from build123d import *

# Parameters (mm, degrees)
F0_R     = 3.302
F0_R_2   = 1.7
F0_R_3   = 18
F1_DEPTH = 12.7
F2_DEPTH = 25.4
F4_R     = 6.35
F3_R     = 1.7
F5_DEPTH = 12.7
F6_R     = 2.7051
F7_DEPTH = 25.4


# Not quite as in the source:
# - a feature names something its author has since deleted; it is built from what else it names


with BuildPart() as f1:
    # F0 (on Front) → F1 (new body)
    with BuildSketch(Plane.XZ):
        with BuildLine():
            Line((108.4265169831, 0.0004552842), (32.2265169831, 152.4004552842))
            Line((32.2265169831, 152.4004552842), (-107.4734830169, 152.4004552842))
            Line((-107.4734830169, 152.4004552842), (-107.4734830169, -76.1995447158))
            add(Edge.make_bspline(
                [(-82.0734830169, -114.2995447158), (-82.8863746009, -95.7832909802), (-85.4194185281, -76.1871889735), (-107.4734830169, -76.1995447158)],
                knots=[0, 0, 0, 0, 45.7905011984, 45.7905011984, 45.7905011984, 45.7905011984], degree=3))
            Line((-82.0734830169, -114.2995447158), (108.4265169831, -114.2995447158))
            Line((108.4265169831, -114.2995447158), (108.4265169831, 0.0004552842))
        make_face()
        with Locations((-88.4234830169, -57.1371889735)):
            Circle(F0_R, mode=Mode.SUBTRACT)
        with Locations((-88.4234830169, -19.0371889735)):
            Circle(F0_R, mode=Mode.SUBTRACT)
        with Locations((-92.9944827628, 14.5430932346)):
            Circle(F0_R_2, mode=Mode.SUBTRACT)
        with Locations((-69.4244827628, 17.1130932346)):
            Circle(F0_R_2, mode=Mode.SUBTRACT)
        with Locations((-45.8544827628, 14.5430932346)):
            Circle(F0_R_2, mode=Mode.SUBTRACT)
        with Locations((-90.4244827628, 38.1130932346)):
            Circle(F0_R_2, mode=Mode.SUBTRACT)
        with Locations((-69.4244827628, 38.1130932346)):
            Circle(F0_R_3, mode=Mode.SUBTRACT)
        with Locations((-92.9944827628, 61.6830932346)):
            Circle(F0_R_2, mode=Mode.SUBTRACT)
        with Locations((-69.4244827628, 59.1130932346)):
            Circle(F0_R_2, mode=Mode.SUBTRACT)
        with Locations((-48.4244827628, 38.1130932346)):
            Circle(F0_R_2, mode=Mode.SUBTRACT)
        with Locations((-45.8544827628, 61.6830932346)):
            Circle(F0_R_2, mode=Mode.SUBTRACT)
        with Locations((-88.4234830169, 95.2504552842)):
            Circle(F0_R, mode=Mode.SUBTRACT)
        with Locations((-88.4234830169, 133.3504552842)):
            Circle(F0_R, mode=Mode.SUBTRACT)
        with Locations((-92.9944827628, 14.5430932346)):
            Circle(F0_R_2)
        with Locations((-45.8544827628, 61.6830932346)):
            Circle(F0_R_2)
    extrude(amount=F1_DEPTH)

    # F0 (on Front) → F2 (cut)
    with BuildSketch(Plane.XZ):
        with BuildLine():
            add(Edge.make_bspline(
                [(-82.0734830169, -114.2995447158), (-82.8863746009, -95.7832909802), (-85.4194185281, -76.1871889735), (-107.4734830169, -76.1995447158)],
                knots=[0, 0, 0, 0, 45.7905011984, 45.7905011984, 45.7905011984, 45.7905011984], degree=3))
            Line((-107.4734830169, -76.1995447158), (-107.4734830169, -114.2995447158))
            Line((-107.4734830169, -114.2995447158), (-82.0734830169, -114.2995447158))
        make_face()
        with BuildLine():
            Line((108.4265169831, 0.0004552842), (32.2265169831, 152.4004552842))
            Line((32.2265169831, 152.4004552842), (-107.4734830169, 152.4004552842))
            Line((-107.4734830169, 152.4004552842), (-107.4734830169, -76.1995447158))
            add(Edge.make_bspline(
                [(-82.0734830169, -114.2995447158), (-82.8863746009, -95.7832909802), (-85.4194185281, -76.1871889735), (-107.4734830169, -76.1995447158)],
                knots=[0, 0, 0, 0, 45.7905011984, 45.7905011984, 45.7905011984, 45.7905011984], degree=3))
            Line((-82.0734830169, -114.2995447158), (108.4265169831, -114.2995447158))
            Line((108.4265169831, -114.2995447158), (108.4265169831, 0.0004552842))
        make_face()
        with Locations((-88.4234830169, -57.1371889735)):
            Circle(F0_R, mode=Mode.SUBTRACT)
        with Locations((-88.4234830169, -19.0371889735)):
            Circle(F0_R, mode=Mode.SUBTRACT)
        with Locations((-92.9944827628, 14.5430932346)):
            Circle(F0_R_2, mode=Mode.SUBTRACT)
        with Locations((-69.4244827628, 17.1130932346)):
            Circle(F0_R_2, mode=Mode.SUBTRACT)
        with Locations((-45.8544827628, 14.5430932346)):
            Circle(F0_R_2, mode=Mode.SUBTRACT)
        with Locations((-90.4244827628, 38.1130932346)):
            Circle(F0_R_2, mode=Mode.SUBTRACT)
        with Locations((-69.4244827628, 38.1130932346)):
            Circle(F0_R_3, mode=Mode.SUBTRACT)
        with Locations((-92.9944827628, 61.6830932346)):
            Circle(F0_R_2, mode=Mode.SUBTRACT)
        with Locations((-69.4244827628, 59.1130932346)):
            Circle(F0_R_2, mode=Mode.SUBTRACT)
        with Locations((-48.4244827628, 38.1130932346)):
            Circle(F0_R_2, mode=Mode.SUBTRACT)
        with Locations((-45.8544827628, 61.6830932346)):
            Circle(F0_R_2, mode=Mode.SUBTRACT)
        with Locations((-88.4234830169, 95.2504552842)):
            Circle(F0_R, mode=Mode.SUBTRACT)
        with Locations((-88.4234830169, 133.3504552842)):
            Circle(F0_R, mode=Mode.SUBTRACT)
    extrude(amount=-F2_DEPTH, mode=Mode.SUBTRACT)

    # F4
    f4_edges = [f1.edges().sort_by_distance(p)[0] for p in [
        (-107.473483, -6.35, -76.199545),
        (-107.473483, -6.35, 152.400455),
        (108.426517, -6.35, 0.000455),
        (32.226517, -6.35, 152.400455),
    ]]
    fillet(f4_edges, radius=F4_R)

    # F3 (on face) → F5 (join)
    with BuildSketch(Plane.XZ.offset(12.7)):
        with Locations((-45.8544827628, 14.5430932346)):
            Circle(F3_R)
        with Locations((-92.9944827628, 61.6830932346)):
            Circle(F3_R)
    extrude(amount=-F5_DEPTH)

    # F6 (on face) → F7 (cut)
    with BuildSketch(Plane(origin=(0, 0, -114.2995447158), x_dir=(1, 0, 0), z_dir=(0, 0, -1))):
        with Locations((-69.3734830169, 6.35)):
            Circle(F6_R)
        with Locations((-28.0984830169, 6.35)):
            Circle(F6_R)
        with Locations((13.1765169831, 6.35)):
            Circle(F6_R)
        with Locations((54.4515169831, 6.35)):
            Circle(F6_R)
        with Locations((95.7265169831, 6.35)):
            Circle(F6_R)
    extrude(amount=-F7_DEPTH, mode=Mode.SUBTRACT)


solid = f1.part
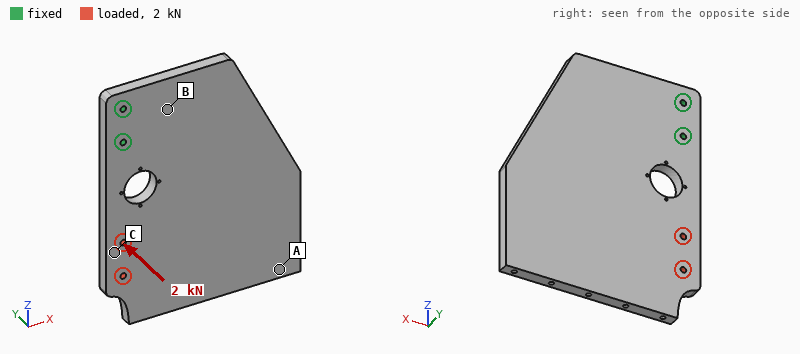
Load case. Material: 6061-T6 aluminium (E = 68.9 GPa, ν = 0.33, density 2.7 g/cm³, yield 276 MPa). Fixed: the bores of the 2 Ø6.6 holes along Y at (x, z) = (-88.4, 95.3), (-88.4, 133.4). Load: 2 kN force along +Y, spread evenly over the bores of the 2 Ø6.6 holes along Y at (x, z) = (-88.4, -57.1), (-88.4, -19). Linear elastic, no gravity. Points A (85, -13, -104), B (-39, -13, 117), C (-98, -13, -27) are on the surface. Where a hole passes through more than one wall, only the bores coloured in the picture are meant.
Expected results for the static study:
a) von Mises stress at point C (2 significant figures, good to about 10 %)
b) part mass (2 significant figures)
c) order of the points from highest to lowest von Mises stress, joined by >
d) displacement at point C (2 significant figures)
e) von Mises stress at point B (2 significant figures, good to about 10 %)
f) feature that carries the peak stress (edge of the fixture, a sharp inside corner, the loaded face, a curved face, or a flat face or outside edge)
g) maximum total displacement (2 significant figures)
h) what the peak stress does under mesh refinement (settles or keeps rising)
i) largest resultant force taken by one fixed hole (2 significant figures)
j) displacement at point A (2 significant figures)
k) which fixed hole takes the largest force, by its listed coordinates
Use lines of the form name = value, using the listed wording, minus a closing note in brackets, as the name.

von Mises stress at point C = 24 MPa
part mass = 1.7 kg
order of the points from highest to lowest von Mises stress, joined by > = B > C > A
displacement at point C = 1.5 mm
von Mises stress at point B = 42 MPa
feature that carries the peak stress = edge of the fixture
maximum total displacement = 2.8 mm
what the peak stress does under mesh refinement = keeps rising
largest resultant force taken by one fixed hole = 5.9 kN
displacement at point A = 2.0 mm
which fixed hole takes the largest force, by its listed coordinates = (-88.4, 95.3)
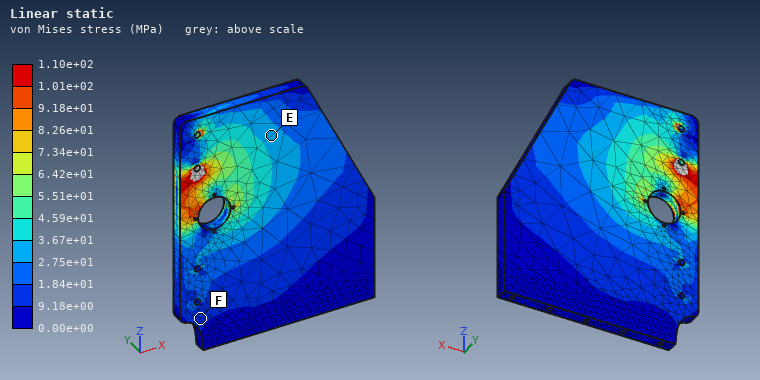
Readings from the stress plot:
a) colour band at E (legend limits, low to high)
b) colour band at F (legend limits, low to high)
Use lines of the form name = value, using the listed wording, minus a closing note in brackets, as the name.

colour band at E = 2.75e+01 to 3.67e+01 MPa
colour band at F = 9.18e+00 to 1.84e+01 MPa
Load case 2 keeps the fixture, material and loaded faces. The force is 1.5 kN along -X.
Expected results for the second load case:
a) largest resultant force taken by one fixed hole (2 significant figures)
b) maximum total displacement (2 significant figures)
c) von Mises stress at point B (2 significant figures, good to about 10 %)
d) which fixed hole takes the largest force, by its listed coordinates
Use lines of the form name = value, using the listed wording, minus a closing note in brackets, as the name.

largest resultant force taken by one fixed hole = 6.2 kN
maximum total displacement = 0.13 mm
von Mises stress at point B = 4.7 MPa
which fixed hole takes the largest force, by its listed coordinates = (-88.4, 95.3)
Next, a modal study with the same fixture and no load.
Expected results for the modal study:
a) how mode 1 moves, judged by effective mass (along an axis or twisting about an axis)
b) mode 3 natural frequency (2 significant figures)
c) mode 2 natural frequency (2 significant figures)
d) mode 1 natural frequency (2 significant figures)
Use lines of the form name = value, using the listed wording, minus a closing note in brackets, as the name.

how mode 1 moves, judged by effective mass = along Y
mode 3 natural frequency = 560 Hz
mode 2 natural frequency = 310 Hz
mode 1 natural frequency = 130 Hz
